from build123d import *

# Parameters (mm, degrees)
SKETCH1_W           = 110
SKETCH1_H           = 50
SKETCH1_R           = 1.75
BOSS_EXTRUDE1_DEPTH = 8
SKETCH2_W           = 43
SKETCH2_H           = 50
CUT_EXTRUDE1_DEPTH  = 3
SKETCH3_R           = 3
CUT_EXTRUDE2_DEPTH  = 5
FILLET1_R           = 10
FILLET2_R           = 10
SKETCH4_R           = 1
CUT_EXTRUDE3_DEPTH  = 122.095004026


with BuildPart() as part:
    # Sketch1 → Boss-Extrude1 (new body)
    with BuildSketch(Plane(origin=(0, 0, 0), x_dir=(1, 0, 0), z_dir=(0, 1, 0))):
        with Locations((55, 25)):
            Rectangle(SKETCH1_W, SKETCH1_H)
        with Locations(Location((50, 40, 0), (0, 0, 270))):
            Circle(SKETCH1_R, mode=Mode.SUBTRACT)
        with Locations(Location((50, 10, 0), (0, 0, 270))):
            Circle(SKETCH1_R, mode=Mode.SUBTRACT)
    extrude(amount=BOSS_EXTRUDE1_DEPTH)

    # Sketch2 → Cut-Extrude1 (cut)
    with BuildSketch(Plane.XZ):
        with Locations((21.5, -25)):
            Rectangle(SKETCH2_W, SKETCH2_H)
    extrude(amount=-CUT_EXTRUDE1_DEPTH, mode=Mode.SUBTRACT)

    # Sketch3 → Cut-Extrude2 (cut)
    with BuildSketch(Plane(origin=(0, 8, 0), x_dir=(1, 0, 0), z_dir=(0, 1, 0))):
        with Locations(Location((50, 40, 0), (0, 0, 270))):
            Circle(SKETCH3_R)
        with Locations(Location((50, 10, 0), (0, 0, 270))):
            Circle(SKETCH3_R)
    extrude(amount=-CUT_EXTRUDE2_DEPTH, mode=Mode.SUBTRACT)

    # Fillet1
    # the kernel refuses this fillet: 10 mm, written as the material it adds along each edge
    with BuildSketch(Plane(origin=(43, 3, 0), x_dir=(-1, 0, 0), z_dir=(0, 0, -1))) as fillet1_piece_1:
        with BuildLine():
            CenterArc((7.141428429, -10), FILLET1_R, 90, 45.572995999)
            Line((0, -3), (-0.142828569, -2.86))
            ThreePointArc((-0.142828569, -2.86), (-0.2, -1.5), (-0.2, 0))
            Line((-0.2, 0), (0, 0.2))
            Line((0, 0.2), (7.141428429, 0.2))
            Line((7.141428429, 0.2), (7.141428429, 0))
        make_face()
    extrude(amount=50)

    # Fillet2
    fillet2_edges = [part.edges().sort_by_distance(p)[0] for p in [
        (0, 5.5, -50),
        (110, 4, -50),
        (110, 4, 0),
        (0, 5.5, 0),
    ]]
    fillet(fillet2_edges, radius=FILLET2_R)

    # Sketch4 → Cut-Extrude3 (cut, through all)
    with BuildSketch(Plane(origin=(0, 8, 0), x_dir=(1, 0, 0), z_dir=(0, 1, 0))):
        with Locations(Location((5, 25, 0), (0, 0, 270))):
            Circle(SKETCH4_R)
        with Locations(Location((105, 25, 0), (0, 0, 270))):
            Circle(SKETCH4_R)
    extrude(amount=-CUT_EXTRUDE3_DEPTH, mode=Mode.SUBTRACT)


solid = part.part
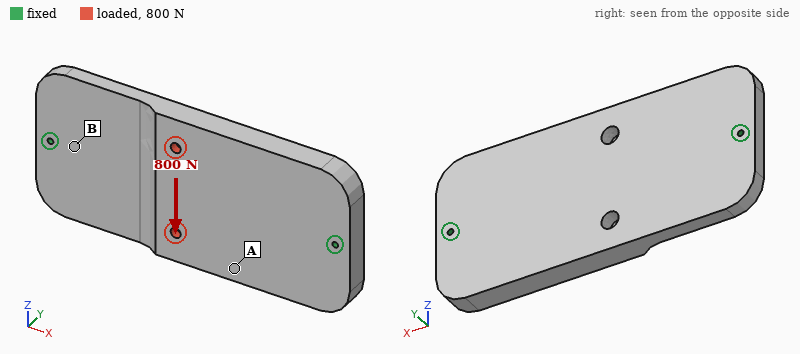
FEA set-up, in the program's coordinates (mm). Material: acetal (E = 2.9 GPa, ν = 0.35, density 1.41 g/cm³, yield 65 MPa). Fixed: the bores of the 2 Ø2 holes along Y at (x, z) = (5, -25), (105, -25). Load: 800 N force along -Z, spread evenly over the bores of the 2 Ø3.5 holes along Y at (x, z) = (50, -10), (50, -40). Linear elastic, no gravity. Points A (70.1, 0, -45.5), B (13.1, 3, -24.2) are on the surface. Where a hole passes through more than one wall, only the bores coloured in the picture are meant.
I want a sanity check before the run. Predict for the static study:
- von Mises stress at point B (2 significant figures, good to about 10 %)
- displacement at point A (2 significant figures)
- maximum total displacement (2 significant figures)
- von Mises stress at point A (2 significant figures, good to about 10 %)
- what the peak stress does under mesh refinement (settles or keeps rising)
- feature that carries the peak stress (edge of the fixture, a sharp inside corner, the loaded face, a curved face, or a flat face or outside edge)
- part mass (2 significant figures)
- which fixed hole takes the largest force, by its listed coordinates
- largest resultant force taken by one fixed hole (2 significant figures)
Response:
8.2 MPa
0.36 mm
0.51 mm
4.3 MPa
keeps rising
edge of the fixture
52 g
(5, -25)
440 N
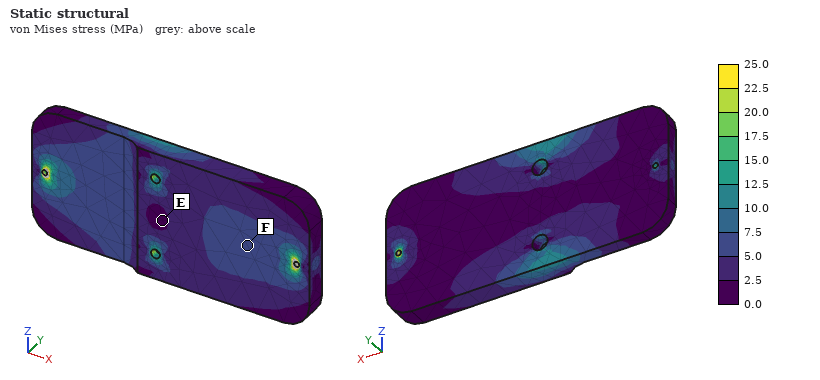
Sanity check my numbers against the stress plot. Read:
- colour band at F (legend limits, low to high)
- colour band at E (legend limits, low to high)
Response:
5.0 to 7.5 MPa
0.0 to 2.5 MPa
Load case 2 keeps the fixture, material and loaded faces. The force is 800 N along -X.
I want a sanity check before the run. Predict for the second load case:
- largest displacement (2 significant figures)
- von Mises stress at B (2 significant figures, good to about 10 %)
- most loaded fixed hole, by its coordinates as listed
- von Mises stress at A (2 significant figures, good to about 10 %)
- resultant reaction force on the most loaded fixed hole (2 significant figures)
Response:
92 µm
4.2 MPa
(105, -25)
2.7 MPa
490 N
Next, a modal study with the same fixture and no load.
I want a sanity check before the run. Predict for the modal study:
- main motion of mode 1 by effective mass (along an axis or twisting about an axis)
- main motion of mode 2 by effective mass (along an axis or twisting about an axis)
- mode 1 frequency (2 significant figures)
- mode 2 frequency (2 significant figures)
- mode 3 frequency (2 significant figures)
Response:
along Y
twisting about X
640 Hz
750 Hz
1700 Hz
